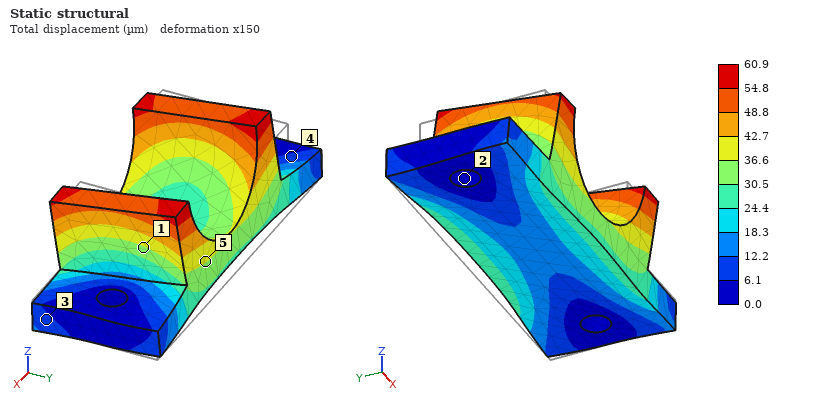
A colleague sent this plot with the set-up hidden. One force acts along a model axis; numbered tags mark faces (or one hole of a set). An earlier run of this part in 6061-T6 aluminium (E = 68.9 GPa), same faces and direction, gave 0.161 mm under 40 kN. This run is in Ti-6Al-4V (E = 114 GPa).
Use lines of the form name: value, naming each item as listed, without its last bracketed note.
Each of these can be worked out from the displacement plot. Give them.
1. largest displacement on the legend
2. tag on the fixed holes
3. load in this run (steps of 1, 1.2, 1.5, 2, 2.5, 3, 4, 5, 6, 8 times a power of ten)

largest displacement on the legend: 60.9 µm
tag on the fixed holes: 2
load in this run: 25 kN
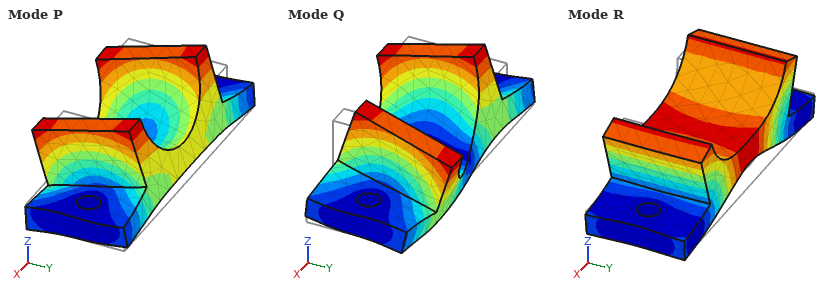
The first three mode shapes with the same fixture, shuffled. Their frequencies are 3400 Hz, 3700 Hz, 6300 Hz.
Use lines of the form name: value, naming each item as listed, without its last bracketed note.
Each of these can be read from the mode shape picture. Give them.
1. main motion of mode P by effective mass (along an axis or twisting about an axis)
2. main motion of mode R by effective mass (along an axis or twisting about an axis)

main motion of mode P by effective mass: along Y
main motion of mode R by effective mass: along Z
